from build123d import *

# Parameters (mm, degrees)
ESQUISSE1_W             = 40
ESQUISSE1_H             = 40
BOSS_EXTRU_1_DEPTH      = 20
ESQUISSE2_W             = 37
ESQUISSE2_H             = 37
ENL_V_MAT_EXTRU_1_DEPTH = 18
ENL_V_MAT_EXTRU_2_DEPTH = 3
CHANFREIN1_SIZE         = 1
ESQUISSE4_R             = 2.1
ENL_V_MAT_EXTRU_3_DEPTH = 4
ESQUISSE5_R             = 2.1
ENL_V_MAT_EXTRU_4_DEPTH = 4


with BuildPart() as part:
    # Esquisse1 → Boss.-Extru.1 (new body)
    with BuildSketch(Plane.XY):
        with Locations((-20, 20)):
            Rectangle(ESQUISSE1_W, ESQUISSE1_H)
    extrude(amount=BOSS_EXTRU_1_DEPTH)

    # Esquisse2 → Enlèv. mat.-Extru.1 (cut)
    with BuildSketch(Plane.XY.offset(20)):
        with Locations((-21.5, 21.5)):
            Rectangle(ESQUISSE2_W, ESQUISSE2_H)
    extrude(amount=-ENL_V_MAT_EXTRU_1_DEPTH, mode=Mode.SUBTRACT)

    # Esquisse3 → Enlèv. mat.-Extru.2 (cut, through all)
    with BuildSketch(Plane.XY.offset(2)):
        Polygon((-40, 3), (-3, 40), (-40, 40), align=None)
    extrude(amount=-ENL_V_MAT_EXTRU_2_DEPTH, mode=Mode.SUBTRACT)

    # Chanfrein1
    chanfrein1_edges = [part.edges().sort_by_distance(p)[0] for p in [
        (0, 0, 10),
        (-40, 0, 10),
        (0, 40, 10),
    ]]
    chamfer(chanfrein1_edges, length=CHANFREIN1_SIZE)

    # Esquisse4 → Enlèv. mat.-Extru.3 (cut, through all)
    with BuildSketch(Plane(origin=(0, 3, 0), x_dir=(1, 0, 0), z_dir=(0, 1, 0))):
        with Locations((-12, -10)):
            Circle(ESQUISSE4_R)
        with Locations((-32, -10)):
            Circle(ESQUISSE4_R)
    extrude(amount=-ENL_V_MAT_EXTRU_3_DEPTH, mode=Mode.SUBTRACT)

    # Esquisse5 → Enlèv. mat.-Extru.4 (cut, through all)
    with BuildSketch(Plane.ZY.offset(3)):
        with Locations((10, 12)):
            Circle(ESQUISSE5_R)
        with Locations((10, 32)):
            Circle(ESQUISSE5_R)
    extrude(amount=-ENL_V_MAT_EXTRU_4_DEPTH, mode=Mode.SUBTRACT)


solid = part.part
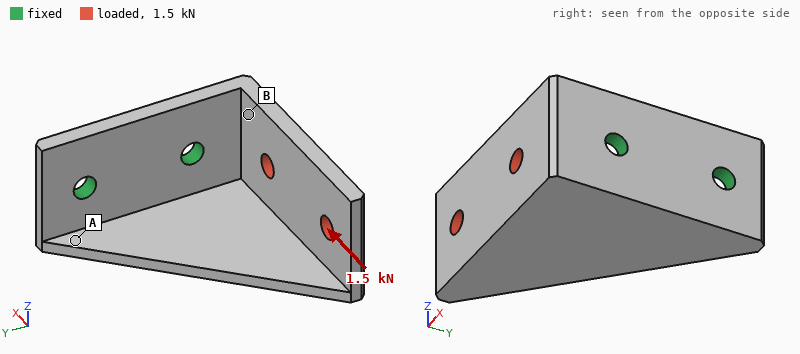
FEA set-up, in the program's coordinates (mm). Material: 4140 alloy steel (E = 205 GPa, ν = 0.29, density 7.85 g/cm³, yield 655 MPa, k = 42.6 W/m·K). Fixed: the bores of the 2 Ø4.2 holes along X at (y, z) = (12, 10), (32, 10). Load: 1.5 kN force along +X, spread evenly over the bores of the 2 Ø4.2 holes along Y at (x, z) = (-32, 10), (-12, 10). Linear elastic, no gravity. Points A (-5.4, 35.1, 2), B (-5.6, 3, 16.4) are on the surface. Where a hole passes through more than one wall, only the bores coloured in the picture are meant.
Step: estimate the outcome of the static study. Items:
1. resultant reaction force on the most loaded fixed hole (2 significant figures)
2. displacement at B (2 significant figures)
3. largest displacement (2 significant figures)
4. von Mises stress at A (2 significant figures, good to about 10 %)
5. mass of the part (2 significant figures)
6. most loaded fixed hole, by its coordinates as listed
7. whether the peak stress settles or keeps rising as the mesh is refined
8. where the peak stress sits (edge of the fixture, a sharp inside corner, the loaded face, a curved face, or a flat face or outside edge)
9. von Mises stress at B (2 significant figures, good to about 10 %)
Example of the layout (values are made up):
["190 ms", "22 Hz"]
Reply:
["1.9 kN", "33 µm", "82 µm", "41 MPa", "45 g", "(12, 10)", "keeps rising", "edge of the fixture", "89 MPa"]
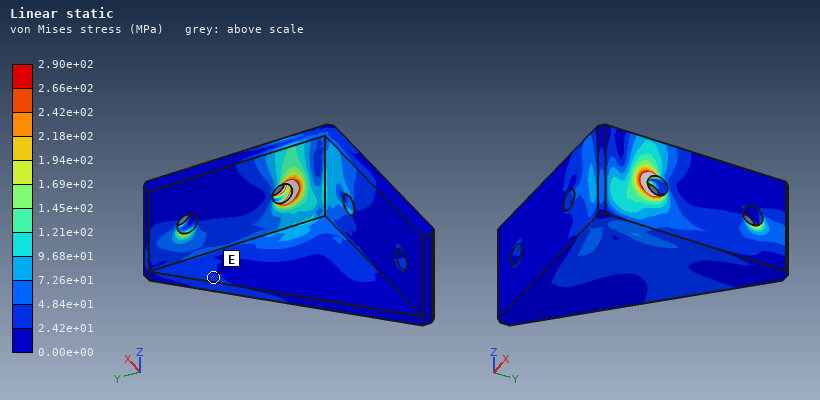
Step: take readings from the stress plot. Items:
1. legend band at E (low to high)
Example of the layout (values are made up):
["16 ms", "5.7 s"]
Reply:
["2.42e+01 to 4.84e+01 MPa"]
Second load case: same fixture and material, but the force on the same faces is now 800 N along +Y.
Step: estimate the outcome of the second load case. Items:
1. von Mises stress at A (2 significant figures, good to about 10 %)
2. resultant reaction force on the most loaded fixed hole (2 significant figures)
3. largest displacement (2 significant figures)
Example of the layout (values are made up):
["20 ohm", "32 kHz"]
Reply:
["61 MPa", "770 N", "0.20 mm"]
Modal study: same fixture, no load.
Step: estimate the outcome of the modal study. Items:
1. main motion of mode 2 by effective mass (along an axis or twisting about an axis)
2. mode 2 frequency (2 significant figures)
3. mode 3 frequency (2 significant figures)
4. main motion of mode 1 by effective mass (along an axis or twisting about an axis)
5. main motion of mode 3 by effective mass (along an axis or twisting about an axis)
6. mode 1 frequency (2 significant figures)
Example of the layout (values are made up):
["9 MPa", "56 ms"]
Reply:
["along Y", "3300 Hz", "7200 Hz", "along Z", "along X", "2200 Hz"]
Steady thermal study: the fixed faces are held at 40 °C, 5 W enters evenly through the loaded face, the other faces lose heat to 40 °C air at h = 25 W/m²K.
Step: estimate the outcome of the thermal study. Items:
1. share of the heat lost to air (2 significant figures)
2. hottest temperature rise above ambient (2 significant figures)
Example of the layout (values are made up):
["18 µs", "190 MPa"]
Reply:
["30 %", "33 K"]
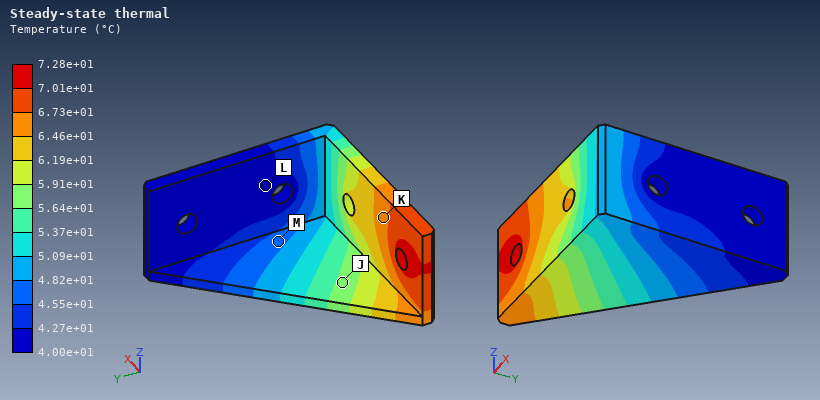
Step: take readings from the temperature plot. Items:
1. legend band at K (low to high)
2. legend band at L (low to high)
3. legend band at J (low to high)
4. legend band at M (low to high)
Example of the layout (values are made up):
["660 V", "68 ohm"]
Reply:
["6.46e+01 to 6.73e+01 °C", "4.00e+01 to 4.27e+01 °C", "5.64e+01 to 5.91e+01 °C", "4.55e+01 to 4.82e+01 °C"]
